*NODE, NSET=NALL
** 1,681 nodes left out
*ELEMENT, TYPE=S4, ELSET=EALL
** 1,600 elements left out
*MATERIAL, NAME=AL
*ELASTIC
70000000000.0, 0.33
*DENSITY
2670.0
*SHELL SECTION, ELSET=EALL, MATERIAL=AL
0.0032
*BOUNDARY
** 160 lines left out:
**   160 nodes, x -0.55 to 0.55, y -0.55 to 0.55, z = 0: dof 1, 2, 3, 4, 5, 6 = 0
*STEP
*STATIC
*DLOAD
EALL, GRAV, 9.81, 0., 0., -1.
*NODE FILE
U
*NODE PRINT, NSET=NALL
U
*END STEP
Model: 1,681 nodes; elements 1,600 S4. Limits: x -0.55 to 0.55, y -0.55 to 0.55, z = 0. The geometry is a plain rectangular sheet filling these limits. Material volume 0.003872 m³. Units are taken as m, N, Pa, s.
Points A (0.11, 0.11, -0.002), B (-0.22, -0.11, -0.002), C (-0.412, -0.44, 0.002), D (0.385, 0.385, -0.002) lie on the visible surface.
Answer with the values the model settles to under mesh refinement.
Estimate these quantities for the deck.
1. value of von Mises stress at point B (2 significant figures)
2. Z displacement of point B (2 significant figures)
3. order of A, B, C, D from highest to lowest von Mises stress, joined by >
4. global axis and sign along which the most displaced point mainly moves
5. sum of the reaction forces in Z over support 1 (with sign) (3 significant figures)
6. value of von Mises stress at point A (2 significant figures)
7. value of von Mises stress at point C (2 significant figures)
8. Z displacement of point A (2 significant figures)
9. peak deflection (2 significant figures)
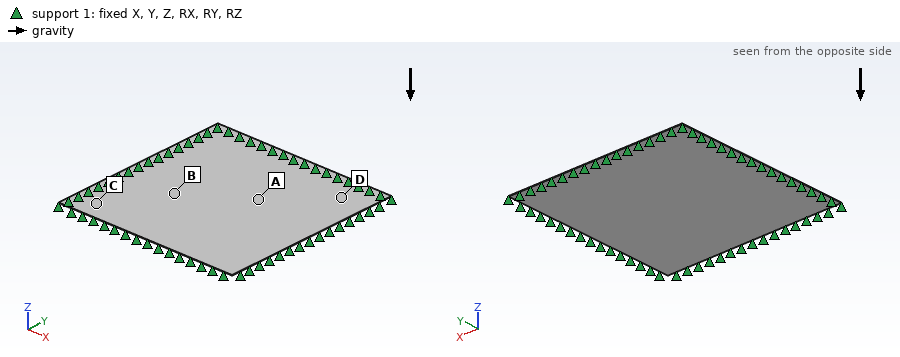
9.5e+05 Pa
-4.9e-04 m
A > B > D > C
-Z
101 N
1.2e+06 Pa
6.9e+05 Pa
-6.2e-04 m
7.1e-04 m
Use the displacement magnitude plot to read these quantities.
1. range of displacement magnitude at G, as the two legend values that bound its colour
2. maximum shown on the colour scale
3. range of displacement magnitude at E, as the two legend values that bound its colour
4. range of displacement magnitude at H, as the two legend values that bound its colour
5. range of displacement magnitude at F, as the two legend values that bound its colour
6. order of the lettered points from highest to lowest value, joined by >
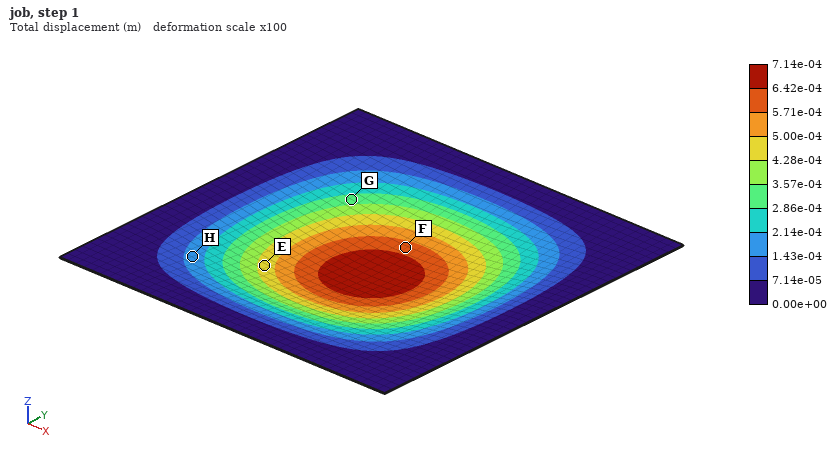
2.86e-04 to 3.57e-04 m
7.14e-04 m
4.28e-04 to 5.00e-04 m
1.43e-04 to 2.14e-04 m
5.71e-04 to 6.42e-04 m
F > E > G > H
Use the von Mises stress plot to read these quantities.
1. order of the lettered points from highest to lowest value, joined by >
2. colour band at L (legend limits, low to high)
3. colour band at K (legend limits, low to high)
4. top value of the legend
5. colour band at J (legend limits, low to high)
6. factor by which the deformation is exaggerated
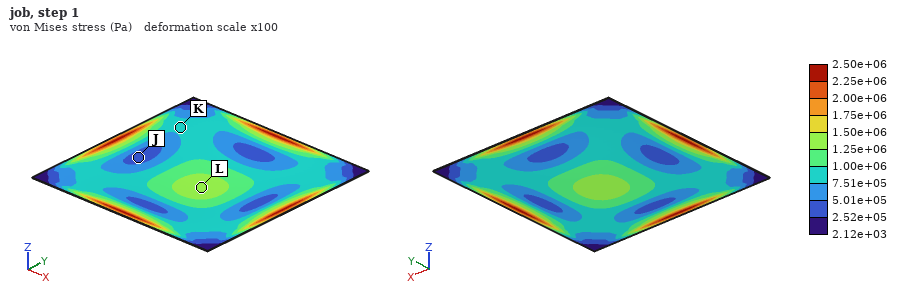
L > K > J
1.25e+06 to 1.50e+06 Pa
7.51e+05 to 1.00e+06 Pa
2.50e+06 Pa
2.52e+05 to 5.01e+05 Pa
100
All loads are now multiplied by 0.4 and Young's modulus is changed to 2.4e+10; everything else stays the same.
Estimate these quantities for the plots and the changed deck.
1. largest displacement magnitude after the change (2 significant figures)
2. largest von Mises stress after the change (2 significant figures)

8.3e-04 m
1.0e+06 Pa
